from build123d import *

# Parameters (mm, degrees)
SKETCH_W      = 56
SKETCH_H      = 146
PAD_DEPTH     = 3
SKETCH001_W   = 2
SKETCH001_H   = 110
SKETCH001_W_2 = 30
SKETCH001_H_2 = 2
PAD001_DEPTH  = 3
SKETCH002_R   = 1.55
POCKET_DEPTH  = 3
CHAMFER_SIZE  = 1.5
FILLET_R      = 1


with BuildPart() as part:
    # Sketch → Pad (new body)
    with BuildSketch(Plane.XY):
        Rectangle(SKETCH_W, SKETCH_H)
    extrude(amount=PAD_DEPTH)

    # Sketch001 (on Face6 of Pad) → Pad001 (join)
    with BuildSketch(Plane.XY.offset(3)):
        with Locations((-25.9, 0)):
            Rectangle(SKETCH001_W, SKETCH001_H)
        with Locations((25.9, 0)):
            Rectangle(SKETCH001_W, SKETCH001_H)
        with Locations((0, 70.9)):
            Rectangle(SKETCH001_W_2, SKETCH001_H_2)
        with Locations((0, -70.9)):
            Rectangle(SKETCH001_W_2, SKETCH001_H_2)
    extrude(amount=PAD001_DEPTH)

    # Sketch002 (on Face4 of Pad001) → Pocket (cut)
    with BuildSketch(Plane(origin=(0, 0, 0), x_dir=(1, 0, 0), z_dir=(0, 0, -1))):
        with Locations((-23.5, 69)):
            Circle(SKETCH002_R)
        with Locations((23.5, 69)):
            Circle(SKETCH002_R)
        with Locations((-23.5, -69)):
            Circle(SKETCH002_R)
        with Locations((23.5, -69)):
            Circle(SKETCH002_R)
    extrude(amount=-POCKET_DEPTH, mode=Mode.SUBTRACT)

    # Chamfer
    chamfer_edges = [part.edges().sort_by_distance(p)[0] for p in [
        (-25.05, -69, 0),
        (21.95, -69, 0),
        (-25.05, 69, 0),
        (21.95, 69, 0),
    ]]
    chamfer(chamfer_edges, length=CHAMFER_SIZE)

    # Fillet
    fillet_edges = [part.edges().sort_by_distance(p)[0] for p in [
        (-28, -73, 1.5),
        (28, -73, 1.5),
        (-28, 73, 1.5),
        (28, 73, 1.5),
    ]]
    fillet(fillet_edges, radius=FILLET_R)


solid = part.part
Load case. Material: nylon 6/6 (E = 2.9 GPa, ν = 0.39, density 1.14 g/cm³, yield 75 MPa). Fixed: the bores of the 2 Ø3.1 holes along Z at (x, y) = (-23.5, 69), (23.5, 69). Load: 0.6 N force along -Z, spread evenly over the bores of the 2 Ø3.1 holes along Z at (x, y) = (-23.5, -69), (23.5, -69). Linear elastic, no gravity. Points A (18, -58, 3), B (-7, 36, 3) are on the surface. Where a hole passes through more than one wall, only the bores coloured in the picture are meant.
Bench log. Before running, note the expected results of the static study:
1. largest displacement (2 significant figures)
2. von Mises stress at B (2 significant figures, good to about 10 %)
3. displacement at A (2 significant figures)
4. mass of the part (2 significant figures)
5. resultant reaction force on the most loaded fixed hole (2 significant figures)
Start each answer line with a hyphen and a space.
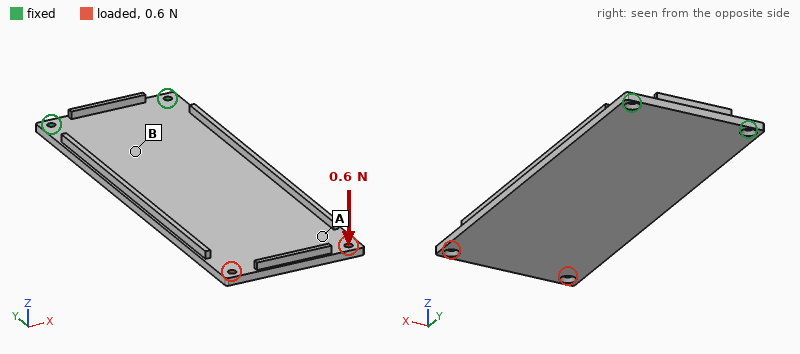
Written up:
- 1.4 mm
- 0.41 MPa
- 1.2 mm
- 30 g
- 0.30 N
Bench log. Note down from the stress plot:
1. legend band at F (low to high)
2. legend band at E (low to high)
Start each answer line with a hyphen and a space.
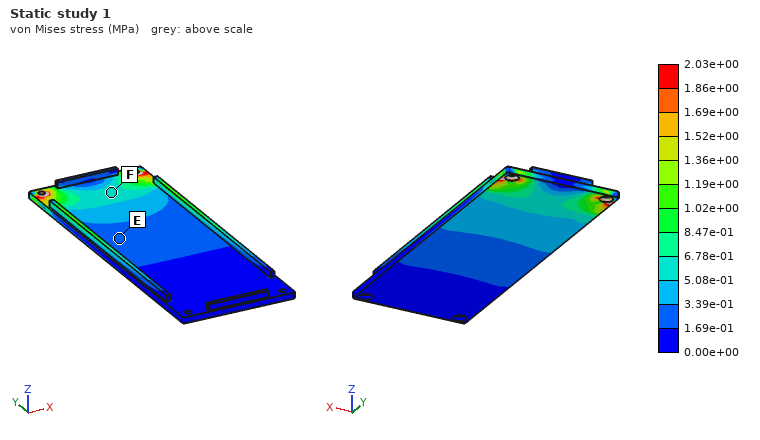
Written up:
- 5.08e-01 to 6.78e-01 MPa
- 1.69e-01 to 3.39e-01 MPa
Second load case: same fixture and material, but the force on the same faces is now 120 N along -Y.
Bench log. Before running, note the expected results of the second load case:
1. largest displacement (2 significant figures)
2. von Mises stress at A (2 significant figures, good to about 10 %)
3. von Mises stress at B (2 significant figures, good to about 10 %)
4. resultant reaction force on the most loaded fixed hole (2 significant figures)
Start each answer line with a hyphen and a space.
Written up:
- 1.5 mm
- 2.1 MPa
- 0.98 MPa
- 62 N
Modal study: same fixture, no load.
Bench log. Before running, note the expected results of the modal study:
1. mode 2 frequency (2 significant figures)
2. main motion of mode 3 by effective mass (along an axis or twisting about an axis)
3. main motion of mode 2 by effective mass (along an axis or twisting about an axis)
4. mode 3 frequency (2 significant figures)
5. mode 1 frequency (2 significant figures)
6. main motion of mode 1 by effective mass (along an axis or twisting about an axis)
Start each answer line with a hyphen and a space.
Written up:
- 190 Hz
- along Z
- twisting about Y
- 270 Hz
- 36 Hz
- along Z
